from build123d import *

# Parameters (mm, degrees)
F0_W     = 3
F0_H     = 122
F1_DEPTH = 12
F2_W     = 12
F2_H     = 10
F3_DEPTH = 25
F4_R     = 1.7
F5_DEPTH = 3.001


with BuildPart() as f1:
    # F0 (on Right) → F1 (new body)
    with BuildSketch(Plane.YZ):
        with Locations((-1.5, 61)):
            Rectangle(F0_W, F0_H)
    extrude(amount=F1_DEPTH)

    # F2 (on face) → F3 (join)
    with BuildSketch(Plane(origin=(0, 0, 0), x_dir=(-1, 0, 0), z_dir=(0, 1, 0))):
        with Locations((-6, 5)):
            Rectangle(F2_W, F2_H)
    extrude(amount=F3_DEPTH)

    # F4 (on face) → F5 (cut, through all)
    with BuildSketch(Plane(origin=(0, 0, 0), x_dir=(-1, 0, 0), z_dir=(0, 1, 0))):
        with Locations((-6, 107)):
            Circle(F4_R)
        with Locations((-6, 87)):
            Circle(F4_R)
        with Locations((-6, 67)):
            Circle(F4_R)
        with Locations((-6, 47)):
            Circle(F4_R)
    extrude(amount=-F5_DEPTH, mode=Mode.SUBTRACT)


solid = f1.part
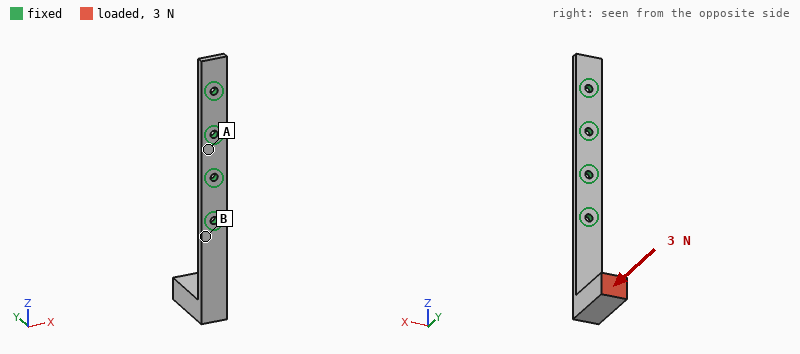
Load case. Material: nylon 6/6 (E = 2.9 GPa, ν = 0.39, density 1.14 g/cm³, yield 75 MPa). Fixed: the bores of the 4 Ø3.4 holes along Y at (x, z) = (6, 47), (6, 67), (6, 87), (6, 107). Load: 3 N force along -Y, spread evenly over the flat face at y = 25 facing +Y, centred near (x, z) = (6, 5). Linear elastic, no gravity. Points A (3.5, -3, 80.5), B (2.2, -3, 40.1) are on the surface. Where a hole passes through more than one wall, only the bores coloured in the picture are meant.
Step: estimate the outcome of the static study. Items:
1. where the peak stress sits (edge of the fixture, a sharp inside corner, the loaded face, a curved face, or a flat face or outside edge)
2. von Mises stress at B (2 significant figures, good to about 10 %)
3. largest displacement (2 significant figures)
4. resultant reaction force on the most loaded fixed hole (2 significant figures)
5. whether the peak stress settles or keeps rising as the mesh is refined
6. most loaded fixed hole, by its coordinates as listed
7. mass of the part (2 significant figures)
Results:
edge of the fixture
5.7 MPa
1.4 mm
3.4 N
keeps rising
(6, 47)
8.3 g
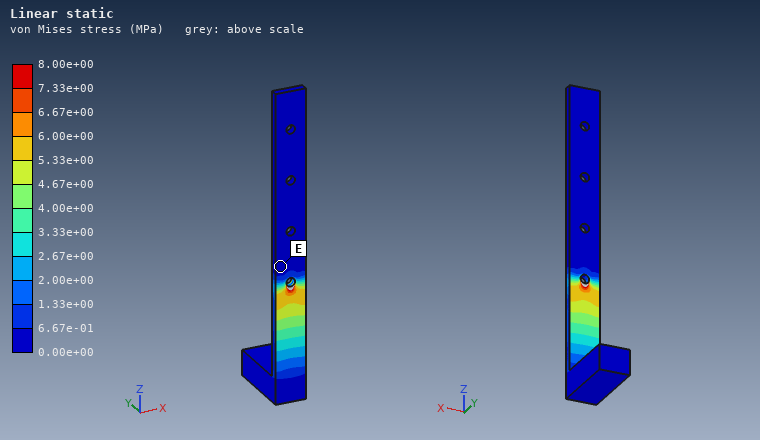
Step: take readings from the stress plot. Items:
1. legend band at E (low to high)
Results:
0.00e+00 to 6.67e-01 MPa
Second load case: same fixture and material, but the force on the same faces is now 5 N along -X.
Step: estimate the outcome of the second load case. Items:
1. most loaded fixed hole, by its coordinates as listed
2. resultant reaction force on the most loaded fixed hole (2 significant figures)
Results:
(6, 47)
11 N
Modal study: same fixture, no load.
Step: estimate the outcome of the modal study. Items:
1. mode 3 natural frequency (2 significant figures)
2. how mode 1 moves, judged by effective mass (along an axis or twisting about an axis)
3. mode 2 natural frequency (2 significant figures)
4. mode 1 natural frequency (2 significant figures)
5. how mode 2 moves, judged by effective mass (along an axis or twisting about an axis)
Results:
600 Hz
along Y
250 Hz
130 Hz
along X
